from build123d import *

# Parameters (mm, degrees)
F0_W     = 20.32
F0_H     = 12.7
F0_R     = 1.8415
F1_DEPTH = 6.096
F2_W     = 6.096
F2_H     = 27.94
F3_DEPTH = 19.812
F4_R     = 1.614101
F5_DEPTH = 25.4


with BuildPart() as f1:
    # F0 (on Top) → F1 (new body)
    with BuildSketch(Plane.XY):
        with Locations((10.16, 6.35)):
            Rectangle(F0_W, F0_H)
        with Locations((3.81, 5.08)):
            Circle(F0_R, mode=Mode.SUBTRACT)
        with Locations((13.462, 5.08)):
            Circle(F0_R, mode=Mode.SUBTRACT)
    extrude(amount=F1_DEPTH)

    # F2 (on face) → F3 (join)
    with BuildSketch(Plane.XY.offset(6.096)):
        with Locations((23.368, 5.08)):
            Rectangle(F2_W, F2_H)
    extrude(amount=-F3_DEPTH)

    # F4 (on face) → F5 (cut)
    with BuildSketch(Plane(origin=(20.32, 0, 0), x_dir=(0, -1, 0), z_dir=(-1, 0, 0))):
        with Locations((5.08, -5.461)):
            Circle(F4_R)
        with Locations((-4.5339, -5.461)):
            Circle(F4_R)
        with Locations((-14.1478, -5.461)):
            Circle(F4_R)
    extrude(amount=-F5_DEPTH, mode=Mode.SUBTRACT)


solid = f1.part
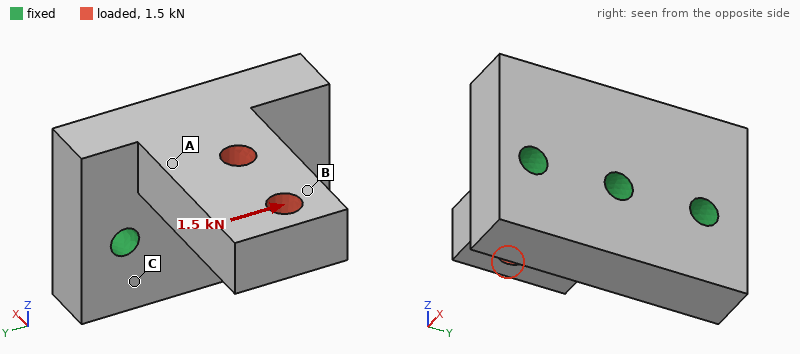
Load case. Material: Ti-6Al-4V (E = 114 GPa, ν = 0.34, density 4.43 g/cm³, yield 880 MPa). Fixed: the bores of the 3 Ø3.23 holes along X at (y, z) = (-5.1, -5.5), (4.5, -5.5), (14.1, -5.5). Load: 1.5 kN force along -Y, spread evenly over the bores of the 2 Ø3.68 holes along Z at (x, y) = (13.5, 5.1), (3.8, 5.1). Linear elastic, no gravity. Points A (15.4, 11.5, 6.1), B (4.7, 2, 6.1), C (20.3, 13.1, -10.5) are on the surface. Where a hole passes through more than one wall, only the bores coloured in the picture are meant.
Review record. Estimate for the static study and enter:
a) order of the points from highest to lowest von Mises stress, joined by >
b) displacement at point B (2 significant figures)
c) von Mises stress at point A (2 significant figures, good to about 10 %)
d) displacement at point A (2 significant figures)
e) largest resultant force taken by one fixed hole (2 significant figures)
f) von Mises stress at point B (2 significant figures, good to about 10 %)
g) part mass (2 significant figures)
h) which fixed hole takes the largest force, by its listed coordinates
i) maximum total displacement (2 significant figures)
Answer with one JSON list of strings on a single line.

["A > B > C", "45 µm", "50 MPa", "19 µm", "1.5 kN", "27 MPa", "21 g", "(14.1, -5.5)", "61 µm"]
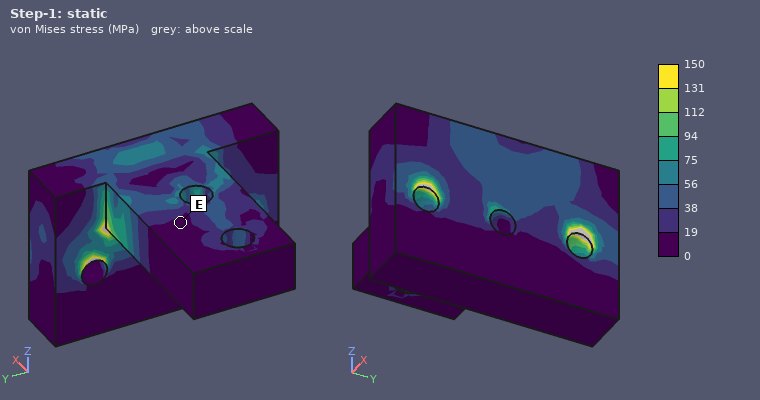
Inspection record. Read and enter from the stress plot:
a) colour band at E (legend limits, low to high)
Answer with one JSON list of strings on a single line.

["0 to 19 MPa"]
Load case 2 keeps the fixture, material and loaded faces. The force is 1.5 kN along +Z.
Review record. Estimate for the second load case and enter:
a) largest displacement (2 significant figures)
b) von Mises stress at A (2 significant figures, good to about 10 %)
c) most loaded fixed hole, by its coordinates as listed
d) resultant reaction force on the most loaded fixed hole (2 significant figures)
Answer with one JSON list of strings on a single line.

["0.19 mm", "160 MPa", "(4.5, -5.5)", "1.1 kN"]
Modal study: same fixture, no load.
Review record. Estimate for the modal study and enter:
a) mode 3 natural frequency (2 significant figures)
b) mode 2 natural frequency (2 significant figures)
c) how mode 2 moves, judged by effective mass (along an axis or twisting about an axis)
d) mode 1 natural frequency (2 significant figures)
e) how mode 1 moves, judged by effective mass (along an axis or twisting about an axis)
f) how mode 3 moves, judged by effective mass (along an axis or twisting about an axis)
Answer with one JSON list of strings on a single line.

["24 kHz", "13 kHz", "along Y", "7500 Hz", "along Z", "along X"]
